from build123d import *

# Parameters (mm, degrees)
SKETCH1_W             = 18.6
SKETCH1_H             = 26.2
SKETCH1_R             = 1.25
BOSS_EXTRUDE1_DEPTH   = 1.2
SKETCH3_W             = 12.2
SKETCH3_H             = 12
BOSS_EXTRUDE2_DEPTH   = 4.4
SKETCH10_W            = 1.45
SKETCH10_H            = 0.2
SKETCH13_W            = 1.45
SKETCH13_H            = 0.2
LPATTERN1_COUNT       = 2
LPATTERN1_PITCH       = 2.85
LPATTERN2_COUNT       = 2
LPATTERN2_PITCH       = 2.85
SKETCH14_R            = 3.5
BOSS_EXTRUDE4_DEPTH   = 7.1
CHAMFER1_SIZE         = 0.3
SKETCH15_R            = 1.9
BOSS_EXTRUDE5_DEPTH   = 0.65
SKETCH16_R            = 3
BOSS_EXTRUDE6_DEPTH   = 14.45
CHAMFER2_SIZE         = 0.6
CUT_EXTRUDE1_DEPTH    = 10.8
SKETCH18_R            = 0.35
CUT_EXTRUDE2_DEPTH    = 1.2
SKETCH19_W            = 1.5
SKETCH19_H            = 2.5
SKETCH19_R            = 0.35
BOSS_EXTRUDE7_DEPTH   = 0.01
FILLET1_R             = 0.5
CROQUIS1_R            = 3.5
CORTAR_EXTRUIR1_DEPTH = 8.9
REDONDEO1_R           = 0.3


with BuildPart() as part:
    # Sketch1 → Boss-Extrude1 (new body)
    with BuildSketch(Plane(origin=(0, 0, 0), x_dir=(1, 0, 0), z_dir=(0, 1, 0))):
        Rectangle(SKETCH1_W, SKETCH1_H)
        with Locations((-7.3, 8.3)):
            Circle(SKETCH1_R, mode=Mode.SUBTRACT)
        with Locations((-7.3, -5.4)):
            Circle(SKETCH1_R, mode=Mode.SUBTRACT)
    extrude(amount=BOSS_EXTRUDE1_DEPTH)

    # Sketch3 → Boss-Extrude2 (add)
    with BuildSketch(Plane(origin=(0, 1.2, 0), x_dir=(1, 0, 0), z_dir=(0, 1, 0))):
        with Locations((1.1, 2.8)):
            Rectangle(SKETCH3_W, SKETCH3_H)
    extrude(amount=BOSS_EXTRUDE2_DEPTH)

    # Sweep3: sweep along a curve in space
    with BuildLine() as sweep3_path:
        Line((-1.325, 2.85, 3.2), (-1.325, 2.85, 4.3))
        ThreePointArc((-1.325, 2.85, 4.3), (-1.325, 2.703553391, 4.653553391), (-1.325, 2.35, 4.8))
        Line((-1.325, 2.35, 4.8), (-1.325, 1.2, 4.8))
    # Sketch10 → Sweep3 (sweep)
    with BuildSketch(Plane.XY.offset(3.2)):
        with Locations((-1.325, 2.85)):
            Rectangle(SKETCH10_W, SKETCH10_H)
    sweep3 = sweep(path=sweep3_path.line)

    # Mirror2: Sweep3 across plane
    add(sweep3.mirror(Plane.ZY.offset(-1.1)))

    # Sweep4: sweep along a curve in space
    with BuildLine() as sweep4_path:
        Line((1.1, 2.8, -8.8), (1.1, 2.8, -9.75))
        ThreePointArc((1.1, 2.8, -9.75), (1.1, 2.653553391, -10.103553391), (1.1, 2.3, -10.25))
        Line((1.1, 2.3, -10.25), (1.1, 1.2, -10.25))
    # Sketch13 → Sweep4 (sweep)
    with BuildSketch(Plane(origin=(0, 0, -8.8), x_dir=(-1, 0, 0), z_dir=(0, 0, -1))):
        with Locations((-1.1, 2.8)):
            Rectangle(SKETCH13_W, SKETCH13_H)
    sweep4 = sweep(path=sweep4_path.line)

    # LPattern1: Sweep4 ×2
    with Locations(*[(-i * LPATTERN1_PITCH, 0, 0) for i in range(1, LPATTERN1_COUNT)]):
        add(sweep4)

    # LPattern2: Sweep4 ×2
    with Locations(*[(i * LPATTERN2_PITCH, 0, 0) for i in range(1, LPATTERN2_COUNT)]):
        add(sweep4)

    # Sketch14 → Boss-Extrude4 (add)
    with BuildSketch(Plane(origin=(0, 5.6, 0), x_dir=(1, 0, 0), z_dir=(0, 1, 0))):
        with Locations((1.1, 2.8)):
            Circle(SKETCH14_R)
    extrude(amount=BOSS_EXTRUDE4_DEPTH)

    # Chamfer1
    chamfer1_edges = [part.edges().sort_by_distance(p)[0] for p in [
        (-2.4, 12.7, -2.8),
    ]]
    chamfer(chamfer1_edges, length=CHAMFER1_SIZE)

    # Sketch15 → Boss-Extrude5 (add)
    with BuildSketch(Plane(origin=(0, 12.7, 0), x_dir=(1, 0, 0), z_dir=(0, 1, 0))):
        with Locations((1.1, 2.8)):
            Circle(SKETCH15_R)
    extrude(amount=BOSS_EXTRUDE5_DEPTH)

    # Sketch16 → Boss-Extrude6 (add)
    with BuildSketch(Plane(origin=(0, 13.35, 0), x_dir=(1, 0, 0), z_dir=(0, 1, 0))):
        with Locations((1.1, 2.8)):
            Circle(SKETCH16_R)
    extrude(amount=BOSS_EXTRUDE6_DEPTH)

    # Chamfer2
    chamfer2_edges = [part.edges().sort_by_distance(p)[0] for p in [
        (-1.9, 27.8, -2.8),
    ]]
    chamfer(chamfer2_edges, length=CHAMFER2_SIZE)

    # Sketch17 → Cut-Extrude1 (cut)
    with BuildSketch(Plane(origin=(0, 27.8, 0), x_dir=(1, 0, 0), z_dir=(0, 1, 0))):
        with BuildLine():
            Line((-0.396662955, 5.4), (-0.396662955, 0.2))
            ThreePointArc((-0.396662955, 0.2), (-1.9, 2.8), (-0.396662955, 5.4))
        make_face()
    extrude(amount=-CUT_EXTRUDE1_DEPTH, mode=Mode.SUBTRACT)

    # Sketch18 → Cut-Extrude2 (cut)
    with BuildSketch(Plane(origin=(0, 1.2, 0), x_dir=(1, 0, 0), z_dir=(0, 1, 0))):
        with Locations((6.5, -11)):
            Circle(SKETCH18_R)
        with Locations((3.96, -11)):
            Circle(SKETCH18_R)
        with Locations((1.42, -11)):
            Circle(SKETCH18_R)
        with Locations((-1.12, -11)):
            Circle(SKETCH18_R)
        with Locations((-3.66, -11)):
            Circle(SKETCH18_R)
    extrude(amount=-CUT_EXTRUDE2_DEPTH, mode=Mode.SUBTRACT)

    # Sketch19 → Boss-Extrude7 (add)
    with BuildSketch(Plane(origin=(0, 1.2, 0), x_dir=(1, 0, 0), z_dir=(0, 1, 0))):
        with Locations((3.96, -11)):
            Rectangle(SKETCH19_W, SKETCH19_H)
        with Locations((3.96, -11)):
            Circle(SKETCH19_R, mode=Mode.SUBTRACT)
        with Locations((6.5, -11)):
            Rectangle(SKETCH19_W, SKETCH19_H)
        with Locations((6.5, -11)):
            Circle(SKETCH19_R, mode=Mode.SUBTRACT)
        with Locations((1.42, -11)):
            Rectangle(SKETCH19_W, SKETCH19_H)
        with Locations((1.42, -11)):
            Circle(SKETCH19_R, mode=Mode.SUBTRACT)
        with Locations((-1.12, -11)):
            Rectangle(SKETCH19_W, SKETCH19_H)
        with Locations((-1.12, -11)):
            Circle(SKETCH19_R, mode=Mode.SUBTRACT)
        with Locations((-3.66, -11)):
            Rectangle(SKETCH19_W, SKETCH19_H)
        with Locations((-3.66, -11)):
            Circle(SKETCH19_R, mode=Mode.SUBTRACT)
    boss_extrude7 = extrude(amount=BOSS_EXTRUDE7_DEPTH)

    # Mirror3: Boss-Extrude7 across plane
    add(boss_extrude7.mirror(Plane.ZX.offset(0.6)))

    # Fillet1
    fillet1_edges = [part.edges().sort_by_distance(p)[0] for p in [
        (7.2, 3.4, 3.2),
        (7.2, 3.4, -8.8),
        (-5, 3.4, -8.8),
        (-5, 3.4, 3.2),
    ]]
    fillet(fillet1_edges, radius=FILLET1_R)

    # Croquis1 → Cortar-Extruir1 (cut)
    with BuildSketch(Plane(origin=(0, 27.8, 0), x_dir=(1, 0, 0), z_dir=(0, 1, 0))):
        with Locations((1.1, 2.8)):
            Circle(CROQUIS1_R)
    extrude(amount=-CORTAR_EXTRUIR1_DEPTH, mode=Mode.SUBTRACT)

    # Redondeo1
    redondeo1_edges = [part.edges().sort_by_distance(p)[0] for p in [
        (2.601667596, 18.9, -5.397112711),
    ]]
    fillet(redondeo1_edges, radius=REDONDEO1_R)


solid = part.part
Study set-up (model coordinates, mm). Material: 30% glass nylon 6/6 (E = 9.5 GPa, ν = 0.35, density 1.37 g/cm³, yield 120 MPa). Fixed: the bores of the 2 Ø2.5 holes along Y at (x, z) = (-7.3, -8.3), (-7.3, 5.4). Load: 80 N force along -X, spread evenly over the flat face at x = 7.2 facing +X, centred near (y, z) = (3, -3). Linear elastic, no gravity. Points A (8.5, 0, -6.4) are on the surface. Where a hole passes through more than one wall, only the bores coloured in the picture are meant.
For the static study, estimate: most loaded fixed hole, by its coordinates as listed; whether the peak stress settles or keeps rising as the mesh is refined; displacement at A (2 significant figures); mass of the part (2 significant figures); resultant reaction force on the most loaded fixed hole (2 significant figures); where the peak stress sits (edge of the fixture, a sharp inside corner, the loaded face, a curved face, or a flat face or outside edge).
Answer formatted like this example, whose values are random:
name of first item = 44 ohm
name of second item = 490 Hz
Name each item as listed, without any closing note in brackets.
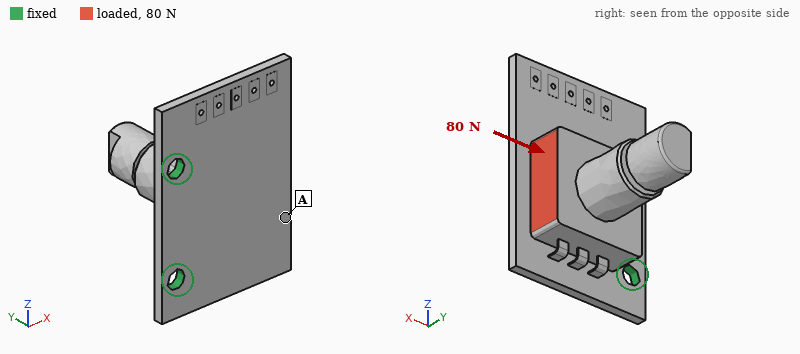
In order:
most loaded fixed hole, by its coordinates as listed = (-7.3, -8.3)
whether the peak stress settles or keeps rising as the mesh is refined = keeps rising
displacement at A = 0.29 mm
mass of the part = 2.3 g
resultant reaction force on the most loaded fixed hole = 49 N
where the peak stress sits = edge of the fixture
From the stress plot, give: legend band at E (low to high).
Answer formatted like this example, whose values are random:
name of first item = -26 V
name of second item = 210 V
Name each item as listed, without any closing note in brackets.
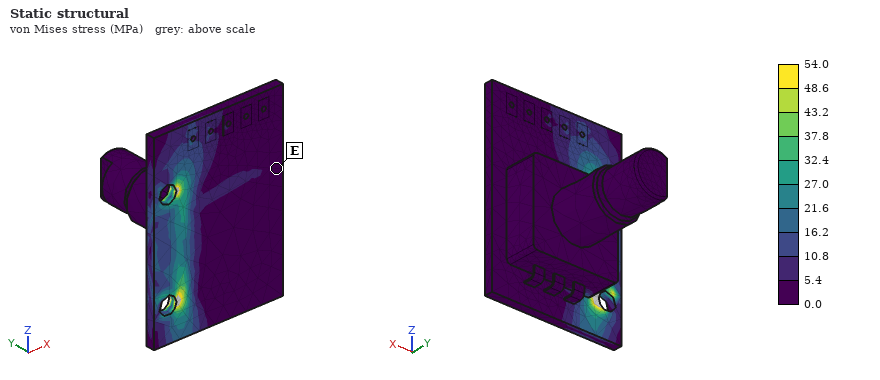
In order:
legend band at E = 0.0 to 5.4 MPa
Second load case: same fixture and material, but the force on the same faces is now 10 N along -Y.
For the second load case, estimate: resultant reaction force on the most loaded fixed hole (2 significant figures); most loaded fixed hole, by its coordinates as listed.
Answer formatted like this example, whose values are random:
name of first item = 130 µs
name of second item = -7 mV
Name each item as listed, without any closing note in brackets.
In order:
resultant reaction force on the most loaded fixed hole = 5.4 N
most loaded fixed hole, by its coordinates as listed = (-7.3, -8.3)
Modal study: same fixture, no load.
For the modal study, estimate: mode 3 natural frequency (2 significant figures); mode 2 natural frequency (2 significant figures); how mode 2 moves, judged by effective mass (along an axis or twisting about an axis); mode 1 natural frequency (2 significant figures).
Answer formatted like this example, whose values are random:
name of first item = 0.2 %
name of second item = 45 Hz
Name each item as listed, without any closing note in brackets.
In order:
mode 3 natural frequency = 6200 Hz
mode 2 natural frequency = 4500 Hz
how mode 2 moves, judged by effective mass = along Z
mode 1 natural frequency = 1100 Hz
